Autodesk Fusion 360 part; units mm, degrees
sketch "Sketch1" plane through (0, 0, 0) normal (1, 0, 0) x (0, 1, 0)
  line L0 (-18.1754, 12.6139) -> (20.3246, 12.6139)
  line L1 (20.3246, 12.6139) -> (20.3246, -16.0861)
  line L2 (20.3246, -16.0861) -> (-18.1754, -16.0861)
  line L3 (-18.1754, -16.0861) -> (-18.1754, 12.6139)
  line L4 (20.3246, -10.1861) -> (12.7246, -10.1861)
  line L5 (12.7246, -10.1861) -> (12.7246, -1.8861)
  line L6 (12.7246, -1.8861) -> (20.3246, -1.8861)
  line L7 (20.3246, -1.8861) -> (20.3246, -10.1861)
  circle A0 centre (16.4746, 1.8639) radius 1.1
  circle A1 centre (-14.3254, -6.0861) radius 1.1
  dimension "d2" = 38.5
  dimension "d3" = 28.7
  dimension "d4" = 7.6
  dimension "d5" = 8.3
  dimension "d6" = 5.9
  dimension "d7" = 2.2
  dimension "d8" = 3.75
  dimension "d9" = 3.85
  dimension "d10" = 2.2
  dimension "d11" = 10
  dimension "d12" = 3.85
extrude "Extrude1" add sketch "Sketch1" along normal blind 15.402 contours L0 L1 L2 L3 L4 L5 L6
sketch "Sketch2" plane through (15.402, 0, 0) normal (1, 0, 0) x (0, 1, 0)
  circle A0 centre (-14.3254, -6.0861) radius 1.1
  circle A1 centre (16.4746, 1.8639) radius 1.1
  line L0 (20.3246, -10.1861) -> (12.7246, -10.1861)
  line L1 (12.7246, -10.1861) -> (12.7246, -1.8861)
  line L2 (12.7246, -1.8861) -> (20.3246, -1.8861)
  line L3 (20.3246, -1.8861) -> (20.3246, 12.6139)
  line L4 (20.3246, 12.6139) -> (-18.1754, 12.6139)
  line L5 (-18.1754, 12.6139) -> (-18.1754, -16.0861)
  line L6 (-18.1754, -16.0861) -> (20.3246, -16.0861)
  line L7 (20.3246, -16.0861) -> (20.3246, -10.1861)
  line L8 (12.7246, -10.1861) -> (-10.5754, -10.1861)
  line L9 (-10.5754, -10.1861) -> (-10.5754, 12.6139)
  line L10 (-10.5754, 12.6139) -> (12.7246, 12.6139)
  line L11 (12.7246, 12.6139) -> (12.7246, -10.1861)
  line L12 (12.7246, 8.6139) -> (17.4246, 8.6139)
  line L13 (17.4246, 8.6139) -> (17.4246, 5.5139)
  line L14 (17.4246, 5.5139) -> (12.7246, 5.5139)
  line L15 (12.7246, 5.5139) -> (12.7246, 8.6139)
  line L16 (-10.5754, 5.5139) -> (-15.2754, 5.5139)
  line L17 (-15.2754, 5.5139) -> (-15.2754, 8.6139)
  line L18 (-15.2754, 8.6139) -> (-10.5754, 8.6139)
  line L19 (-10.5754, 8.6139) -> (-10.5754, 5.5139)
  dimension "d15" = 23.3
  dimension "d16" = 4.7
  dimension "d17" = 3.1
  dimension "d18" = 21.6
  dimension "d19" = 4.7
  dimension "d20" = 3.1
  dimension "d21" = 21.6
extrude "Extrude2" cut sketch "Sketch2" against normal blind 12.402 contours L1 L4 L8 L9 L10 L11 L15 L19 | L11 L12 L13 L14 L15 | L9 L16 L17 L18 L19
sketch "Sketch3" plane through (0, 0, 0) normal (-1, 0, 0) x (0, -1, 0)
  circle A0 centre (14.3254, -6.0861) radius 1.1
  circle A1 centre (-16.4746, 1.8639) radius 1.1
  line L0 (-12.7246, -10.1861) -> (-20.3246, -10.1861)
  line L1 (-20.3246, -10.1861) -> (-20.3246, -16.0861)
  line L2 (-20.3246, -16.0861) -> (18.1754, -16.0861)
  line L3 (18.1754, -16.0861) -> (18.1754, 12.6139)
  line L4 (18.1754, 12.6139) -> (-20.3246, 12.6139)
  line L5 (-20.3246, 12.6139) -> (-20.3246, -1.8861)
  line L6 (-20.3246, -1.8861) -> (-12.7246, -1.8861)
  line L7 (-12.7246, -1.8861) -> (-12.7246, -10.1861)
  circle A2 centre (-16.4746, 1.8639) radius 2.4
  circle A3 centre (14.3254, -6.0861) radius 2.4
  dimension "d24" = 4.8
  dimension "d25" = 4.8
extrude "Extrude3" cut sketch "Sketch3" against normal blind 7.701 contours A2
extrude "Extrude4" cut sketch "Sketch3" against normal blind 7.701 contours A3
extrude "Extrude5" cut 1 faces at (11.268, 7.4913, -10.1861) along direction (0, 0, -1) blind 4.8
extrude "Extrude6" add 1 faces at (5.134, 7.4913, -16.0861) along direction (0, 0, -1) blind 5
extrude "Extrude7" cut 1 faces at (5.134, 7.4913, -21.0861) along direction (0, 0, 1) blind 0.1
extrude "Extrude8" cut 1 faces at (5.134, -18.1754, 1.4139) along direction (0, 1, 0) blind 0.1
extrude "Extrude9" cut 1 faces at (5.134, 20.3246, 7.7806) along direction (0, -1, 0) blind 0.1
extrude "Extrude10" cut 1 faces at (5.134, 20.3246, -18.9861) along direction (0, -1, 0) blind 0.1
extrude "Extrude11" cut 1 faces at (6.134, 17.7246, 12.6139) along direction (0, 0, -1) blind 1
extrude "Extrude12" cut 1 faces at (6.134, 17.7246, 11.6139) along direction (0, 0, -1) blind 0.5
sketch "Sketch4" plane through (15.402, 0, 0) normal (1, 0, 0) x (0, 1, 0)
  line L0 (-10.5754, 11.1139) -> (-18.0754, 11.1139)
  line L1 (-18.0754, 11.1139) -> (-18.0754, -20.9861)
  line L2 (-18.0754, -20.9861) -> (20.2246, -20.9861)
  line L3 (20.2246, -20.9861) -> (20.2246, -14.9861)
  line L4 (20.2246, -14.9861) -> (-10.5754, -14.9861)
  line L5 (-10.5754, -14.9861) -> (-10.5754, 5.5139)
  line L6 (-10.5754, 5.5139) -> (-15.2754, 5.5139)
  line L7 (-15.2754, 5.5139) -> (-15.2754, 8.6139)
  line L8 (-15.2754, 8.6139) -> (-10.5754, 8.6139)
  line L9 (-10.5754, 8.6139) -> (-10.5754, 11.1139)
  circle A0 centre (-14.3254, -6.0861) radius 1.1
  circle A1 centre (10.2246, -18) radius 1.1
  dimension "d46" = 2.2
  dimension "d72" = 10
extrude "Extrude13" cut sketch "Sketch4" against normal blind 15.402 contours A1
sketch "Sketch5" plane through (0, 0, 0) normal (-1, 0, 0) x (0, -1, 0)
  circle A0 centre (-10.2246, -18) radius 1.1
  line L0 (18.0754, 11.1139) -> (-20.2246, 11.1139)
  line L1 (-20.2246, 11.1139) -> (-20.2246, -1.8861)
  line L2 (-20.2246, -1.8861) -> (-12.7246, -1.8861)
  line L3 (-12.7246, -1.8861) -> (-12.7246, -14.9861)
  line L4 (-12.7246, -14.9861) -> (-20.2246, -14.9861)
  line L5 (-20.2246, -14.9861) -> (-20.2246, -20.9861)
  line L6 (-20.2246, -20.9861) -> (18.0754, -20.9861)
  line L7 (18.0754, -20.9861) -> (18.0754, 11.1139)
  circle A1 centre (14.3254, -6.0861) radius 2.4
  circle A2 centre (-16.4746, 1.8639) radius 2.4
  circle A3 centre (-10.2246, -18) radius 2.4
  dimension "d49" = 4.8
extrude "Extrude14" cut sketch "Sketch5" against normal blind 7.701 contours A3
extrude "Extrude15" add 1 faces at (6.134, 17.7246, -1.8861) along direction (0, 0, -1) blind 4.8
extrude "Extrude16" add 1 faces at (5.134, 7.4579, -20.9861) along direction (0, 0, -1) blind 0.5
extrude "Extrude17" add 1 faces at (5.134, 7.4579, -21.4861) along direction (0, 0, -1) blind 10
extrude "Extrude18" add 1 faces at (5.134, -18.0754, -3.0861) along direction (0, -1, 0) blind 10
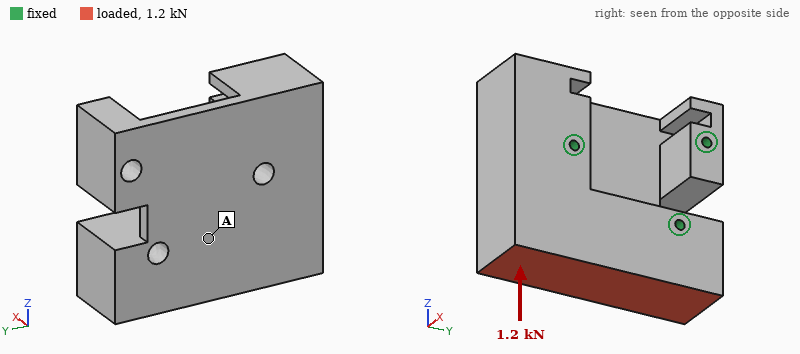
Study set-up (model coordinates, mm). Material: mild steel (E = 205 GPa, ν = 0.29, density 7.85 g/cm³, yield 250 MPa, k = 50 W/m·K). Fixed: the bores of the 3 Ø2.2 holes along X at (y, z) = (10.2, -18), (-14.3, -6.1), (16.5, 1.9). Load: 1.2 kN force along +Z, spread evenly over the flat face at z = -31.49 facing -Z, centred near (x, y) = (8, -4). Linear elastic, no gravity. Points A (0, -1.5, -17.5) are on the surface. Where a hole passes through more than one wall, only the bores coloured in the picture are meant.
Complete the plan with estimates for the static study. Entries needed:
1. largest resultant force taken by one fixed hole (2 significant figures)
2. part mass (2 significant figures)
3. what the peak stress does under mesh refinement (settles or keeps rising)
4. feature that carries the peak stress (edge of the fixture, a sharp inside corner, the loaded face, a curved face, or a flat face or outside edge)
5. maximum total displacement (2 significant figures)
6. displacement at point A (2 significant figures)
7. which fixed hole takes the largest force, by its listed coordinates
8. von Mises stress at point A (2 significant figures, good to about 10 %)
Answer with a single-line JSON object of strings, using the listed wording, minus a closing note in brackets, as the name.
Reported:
{"largest resultant force taken by one fixed hole": "640 N", "part mass": "180 g", "what the peak stress does under mesh refinement": "keeps rising", "feature that carries the peak stress": "edge of the fixture", "maximum total displacement": "2.2 µm", "displacement at point A": "1.0 µm", "which fixed hole takes the largest force, by its listed coordinates": "(-14.3, -6.1)", "von Mises stress at point A": "3.0 MPa"}
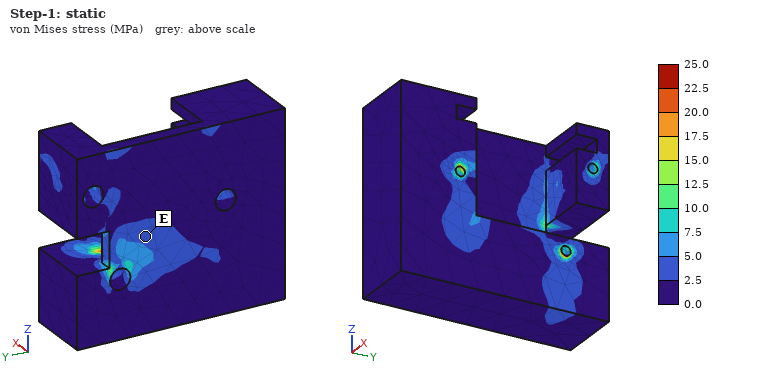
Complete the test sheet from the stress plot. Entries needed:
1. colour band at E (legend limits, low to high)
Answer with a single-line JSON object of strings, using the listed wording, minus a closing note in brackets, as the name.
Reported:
{"colour band at E": "2.5 to 5.0 MPa"}
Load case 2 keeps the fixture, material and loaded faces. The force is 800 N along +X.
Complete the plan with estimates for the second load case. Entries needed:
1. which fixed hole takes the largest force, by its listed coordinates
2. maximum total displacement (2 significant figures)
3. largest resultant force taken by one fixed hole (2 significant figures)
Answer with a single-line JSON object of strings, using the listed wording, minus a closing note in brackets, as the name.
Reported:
{"which fixed hole takes the largest force, by its listed coordinates": "(10.2, -18)", "maximum total displacement": "8.7 µm", "largest resultant force taken by one fixed hole": "680 N"}
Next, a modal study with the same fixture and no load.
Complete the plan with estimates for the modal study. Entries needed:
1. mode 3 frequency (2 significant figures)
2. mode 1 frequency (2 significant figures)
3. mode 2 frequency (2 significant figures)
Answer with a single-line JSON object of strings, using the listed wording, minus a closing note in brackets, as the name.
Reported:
{"mode 3 frequency": "14 kHz", "mode 1 frequency": "7200 Hz", "mode 2 frequency": "14 kHz"}
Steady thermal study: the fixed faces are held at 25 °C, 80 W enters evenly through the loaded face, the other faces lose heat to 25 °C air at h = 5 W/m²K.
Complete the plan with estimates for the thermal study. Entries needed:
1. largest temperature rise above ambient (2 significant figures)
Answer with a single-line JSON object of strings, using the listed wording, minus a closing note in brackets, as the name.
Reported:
{"largest temperature rise above ambient": "76 K"}
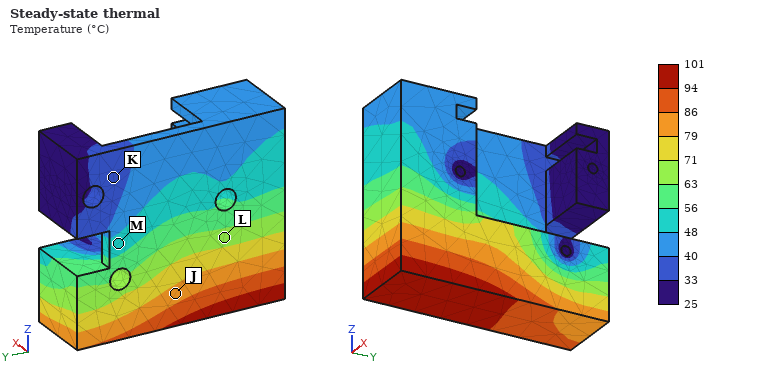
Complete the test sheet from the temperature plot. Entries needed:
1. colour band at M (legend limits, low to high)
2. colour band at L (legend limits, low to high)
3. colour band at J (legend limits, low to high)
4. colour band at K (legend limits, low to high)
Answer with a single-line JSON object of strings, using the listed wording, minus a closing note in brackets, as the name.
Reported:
{"colour band at M": "48 to 56 °C", "colour band at L": "63 to 71 °C", "colour band at J": "79 to 86 °C", "colour band at K": "33 to 40 °C"}
